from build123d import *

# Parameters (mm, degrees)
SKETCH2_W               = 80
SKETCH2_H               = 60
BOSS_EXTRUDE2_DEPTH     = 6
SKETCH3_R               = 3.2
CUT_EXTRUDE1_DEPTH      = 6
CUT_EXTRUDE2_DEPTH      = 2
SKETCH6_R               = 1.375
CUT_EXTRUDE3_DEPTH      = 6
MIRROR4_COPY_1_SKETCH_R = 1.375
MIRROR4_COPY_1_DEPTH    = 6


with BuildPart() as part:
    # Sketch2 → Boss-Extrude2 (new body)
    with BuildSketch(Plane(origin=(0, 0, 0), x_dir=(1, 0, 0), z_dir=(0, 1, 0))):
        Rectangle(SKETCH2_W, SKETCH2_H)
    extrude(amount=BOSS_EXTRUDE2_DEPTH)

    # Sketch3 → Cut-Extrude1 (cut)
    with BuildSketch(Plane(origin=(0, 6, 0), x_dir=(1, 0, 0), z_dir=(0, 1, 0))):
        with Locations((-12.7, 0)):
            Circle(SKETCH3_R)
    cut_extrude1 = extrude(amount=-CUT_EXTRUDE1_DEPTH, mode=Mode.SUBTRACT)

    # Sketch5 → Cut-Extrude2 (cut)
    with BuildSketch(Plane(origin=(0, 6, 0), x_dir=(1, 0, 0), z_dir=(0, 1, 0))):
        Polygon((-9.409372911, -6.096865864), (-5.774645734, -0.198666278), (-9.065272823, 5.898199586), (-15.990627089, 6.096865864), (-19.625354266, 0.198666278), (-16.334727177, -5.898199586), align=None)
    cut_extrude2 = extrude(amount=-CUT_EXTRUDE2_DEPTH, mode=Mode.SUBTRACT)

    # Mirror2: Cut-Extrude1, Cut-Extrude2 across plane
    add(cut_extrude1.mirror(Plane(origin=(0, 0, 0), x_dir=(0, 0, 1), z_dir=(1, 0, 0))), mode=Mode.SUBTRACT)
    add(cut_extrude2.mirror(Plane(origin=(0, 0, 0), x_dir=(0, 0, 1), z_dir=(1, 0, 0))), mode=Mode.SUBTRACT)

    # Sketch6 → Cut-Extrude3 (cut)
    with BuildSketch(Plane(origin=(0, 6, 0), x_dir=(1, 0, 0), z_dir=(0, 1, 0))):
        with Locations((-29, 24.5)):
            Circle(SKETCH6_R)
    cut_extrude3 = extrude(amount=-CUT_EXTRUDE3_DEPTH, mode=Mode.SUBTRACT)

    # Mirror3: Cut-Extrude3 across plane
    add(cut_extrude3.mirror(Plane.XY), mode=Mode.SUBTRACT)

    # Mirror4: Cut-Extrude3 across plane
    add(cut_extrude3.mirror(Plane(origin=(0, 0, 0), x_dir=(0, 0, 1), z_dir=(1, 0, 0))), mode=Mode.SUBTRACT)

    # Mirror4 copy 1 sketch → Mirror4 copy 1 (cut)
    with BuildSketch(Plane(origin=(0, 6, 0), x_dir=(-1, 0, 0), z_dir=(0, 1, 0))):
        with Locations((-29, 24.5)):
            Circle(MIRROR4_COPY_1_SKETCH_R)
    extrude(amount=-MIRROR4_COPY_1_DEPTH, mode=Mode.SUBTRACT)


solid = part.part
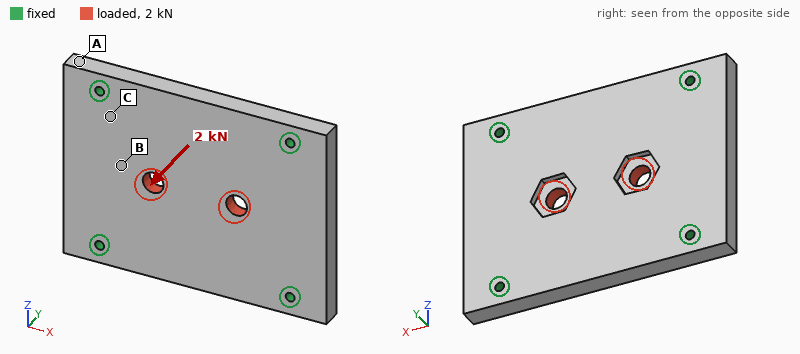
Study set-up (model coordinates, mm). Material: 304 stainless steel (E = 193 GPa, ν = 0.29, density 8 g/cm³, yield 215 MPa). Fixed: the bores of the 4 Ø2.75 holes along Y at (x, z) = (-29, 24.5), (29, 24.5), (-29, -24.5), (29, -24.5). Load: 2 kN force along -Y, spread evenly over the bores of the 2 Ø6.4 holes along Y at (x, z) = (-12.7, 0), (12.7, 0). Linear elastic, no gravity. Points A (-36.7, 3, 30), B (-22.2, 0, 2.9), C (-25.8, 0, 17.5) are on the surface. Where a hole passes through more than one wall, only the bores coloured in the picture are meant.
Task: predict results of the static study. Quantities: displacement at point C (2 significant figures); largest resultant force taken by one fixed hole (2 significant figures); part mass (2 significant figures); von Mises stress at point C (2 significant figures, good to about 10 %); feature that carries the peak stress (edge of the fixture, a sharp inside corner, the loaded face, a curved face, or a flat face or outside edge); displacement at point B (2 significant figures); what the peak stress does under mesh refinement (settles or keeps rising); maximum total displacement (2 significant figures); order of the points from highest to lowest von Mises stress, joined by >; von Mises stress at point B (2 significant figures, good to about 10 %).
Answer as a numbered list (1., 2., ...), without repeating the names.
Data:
1. 4.4 µm
2. 510 N
3. 220 g
4. 22 MPa
5. edge of the fixture
6. 13 µm
7. keeps rising
8. 24 µm
9. B > C > A
10. 34 MPa
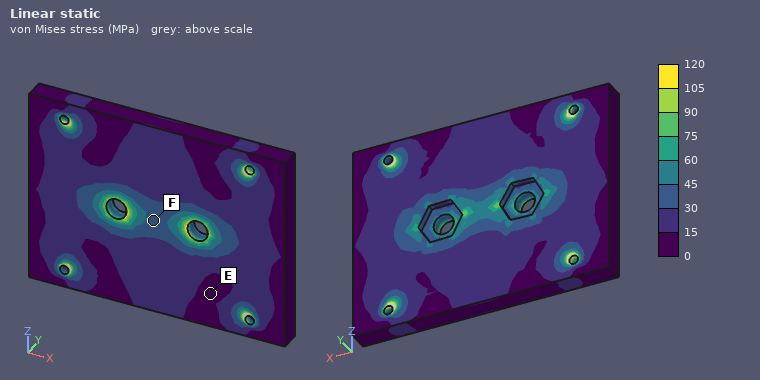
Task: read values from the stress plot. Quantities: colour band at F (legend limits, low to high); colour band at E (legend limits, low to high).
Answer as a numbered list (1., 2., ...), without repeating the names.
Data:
1. 30 to 45 MPa
2. 0 to 15 MPa
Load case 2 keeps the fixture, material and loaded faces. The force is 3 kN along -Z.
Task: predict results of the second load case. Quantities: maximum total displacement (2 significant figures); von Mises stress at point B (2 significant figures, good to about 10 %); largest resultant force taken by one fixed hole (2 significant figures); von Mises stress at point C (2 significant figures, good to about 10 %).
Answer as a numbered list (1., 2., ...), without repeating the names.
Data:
1. 2.2 µm
2. 8.4 MPa
3. 830 N
4. 11 MPa
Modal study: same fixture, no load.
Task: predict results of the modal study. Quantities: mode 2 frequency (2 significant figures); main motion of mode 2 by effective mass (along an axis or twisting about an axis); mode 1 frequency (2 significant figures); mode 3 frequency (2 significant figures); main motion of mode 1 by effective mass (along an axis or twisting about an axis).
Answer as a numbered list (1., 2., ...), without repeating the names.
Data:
1. 9200 Hz
2. twisting about X
3. 6000 Hz
4. 10 kHz
5. along Y
